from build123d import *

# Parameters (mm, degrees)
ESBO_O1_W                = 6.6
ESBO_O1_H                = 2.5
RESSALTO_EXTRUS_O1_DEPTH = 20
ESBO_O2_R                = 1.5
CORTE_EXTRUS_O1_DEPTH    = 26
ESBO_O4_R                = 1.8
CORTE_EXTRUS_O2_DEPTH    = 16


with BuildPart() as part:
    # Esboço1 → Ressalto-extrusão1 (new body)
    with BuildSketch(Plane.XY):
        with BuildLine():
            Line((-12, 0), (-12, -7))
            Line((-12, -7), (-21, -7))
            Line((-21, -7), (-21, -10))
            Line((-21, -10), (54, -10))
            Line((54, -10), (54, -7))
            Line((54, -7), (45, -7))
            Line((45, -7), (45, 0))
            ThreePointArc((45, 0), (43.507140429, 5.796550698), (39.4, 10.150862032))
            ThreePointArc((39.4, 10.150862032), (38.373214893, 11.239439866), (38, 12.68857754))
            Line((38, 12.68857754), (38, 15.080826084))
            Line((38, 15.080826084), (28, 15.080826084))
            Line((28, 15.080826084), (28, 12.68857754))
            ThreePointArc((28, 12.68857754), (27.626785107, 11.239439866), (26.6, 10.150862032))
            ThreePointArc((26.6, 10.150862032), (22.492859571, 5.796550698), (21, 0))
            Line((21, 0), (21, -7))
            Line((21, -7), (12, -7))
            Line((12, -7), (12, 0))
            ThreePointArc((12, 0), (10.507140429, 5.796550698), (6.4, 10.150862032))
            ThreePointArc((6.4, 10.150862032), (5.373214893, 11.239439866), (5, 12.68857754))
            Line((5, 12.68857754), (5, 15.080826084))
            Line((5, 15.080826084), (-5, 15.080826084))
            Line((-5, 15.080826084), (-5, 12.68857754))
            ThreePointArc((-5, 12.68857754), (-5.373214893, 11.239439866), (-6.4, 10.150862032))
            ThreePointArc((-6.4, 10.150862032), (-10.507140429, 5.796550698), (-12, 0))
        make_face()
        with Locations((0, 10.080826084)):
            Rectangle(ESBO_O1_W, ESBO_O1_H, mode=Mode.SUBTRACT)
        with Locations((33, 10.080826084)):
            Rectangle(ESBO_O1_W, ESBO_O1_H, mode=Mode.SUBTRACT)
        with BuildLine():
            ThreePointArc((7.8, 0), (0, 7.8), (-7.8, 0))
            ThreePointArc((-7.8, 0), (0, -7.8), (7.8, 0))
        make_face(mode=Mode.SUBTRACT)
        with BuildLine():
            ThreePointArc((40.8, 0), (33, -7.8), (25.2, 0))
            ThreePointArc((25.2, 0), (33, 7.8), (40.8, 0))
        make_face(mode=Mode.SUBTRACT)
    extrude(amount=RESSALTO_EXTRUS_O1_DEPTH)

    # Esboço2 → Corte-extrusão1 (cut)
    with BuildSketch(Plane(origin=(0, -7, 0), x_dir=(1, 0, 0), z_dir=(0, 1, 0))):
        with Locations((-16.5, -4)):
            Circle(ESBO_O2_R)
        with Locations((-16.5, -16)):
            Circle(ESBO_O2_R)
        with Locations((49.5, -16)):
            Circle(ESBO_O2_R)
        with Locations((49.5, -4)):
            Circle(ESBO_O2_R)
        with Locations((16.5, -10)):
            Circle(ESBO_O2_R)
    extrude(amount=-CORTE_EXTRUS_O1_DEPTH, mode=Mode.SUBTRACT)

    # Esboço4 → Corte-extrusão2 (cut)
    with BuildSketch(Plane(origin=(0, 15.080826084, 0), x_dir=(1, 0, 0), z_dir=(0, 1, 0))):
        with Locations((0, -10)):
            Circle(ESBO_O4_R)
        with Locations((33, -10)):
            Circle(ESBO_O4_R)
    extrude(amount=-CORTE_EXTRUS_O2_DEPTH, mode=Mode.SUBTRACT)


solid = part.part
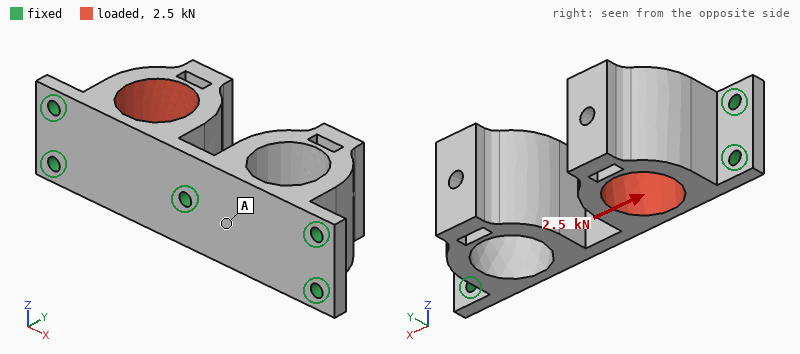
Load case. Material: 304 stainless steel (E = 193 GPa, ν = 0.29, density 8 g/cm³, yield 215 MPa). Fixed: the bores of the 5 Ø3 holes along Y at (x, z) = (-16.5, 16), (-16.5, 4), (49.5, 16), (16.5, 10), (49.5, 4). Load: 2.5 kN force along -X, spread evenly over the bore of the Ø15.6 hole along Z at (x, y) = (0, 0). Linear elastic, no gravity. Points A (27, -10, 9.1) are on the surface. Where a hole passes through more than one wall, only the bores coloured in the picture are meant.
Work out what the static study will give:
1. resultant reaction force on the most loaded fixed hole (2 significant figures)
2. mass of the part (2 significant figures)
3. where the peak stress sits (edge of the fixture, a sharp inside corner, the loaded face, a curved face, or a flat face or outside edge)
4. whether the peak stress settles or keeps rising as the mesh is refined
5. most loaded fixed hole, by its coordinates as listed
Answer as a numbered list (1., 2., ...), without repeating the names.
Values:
1. 1.2 kN
2. 110 g
3. edge of the fixture
4. keeps rising
5. (16.5, 10)
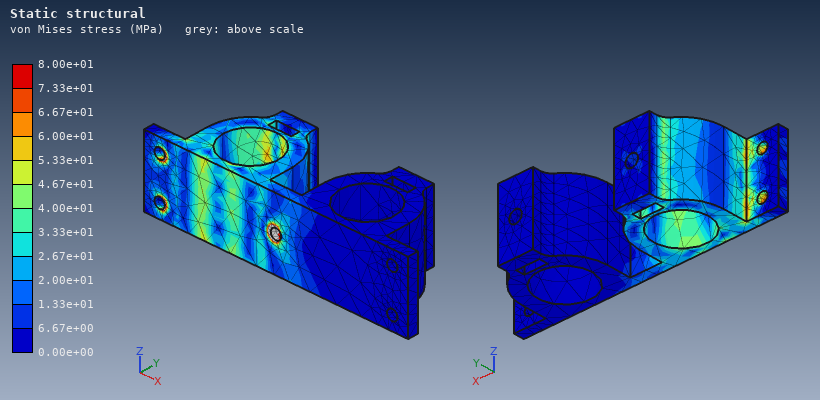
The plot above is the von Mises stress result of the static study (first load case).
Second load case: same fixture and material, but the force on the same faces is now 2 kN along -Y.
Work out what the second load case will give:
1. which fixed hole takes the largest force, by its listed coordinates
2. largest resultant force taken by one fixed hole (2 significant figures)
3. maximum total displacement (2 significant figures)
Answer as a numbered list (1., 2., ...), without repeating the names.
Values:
1. (16.5, 10)
2. 1.0 kN
3. 8.7 µm
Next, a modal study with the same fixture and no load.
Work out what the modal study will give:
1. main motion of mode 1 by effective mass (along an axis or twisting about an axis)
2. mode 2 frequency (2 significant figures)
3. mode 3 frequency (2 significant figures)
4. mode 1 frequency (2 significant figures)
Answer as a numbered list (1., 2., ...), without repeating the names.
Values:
1. along Z
2. 6800 Hz
3. 11 kHz
4. 6000 Hz
